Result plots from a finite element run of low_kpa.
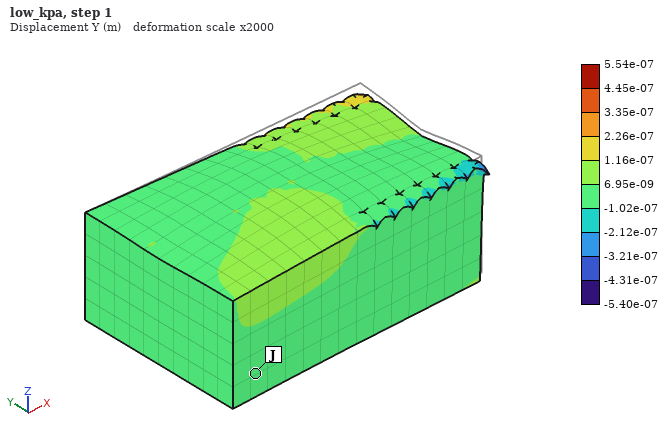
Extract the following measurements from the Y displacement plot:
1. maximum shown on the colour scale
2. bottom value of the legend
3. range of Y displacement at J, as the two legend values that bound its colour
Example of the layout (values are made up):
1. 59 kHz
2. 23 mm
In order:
1. 5.54e-07 m
2. -5.40e-07 m
3. -1.02e-07 to 6.95e-09 m
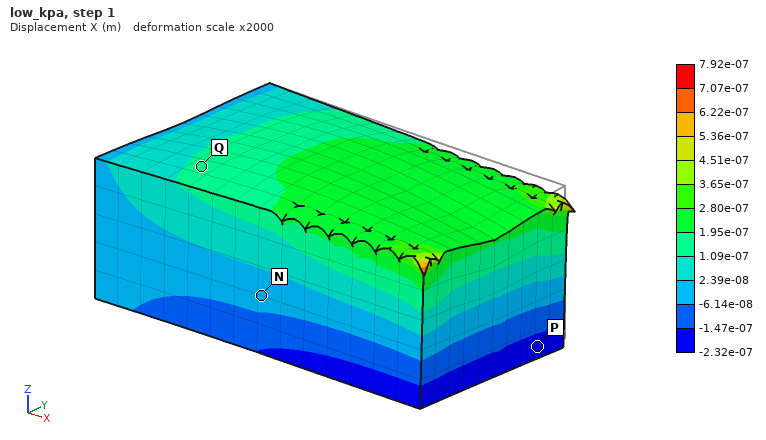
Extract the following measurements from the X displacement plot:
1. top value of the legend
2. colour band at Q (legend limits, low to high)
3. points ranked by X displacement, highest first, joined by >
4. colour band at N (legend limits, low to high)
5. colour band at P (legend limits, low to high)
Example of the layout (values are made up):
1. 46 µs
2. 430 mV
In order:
1. 7.92e-07 m
2. 1.09e-07 to 1.95e-07 m
3. Q > N > P
4. -6.14e-08 to 2.39e-08 m
5. -2.32e-07 to -1.47e-07 m
